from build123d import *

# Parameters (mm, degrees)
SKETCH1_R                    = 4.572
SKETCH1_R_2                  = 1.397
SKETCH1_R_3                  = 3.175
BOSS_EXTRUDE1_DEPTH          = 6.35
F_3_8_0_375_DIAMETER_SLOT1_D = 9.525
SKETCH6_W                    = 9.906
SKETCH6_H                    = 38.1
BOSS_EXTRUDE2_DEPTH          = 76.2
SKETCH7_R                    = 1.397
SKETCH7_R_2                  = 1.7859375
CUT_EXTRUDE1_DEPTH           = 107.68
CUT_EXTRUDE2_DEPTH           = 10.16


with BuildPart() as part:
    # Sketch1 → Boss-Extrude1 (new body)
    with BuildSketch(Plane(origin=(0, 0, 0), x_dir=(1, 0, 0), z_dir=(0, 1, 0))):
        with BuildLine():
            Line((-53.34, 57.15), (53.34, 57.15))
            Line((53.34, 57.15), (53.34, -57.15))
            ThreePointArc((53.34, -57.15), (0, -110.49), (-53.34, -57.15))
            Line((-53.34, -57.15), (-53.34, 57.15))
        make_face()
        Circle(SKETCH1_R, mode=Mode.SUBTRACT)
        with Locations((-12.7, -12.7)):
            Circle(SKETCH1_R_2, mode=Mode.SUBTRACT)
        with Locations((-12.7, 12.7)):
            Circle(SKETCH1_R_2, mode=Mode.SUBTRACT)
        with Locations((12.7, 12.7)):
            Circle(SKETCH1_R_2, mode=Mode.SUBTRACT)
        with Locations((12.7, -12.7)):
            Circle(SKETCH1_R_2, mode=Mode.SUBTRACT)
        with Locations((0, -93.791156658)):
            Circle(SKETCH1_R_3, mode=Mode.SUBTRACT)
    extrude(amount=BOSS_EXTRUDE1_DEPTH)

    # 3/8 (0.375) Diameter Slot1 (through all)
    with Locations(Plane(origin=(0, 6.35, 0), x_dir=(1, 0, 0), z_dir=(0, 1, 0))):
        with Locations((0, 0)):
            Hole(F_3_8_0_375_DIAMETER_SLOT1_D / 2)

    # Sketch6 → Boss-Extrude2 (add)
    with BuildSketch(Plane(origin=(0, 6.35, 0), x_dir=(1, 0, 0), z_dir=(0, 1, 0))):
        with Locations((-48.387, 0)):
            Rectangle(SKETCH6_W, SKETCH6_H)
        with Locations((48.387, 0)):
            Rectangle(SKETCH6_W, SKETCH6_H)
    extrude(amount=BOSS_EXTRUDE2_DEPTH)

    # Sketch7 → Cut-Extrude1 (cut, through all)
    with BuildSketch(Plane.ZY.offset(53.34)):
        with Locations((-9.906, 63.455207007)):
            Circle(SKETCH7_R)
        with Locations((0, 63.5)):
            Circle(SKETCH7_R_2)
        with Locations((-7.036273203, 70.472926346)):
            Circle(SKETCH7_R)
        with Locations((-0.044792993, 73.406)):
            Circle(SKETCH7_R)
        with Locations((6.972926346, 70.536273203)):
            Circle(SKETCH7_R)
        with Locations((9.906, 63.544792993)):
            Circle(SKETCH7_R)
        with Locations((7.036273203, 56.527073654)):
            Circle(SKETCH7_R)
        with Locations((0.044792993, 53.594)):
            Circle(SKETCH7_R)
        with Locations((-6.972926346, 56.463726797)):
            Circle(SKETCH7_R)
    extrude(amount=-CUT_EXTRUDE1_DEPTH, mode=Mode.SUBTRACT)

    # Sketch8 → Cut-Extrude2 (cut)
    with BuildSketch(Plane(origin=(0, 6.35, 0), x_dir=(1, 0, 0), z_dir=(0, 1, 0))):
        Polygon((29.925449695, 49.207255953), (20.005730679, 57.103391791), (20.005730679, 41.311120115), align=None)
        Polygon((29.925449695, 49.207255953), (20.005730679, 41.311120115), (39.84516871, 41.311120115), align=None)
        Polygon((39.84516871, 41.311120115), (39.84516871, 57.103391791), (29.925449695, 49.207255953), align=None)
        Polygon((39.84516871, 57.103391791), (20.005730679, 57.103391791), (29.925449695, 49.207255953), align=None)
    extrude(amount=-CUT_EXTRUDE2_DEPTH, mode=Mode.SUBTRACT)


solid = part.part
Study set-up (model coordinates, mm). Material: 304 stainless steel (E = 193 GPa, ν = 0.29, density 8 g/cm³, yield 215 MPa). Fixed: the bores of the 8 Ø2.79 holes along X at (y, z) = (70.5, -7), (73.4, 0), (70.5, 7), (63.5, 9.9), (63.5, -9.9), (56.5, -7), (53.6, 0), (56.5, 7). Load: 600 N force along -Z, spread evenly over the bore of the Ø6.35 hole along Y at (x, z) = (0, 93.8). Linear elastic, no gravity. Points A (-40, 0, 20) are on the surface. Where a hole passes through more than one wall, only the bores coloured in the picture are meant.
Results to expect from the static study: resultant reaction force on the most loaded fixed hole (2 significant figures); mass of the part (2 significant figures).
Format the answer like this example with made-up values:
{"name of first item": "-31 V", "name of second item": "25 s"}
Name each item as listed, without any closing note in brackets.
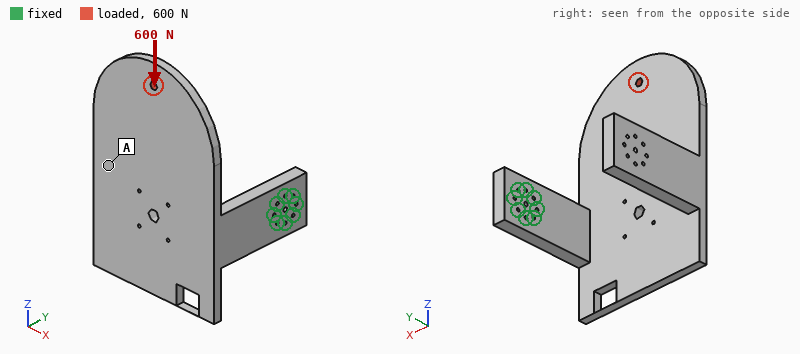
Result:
{"resultant reaction force on the most loaded fixed hole": "1.0 kN", "mass of the part": "1.3 kg"}
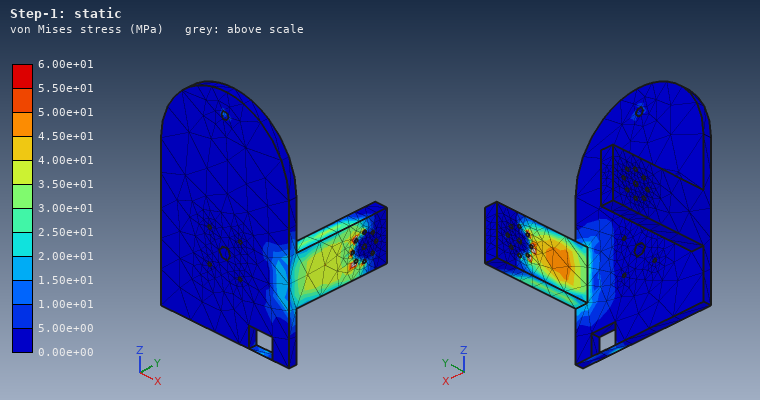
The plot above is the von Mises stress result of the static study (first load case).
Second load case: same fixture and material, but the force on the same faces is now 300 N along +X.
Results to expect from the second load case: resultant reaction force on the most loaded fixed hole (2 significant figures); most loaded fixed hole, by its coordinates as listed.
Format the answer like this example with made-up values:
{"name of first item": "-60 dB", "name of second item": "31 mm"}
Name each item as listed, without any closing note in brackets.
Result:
{"resultant reaction force on the most loaded fixed hole": "840 N", "most loaded fixed hole, by its coordinates as listed": "(56.5, 7)"}
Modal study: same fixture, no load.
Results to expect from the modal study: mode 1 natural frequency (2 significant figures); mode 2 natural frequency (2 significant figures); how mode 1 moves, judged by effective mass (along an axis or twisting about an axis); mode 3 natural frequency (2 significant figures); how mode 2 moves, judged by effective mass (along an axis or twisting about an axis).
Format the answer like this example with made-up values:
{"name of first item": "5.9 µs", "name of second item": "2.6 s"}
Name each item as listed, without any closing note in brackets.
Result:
{"mode 1 natural frequency": "170 Hz", "mode 2 natural frequency": "230 Hz", "how mode 1 moves, judged by effective mass": "along Y", "mode 3 natural frequency": "370 Hz", "how mode 2 moves, judged by effective mass": "along Z"}
